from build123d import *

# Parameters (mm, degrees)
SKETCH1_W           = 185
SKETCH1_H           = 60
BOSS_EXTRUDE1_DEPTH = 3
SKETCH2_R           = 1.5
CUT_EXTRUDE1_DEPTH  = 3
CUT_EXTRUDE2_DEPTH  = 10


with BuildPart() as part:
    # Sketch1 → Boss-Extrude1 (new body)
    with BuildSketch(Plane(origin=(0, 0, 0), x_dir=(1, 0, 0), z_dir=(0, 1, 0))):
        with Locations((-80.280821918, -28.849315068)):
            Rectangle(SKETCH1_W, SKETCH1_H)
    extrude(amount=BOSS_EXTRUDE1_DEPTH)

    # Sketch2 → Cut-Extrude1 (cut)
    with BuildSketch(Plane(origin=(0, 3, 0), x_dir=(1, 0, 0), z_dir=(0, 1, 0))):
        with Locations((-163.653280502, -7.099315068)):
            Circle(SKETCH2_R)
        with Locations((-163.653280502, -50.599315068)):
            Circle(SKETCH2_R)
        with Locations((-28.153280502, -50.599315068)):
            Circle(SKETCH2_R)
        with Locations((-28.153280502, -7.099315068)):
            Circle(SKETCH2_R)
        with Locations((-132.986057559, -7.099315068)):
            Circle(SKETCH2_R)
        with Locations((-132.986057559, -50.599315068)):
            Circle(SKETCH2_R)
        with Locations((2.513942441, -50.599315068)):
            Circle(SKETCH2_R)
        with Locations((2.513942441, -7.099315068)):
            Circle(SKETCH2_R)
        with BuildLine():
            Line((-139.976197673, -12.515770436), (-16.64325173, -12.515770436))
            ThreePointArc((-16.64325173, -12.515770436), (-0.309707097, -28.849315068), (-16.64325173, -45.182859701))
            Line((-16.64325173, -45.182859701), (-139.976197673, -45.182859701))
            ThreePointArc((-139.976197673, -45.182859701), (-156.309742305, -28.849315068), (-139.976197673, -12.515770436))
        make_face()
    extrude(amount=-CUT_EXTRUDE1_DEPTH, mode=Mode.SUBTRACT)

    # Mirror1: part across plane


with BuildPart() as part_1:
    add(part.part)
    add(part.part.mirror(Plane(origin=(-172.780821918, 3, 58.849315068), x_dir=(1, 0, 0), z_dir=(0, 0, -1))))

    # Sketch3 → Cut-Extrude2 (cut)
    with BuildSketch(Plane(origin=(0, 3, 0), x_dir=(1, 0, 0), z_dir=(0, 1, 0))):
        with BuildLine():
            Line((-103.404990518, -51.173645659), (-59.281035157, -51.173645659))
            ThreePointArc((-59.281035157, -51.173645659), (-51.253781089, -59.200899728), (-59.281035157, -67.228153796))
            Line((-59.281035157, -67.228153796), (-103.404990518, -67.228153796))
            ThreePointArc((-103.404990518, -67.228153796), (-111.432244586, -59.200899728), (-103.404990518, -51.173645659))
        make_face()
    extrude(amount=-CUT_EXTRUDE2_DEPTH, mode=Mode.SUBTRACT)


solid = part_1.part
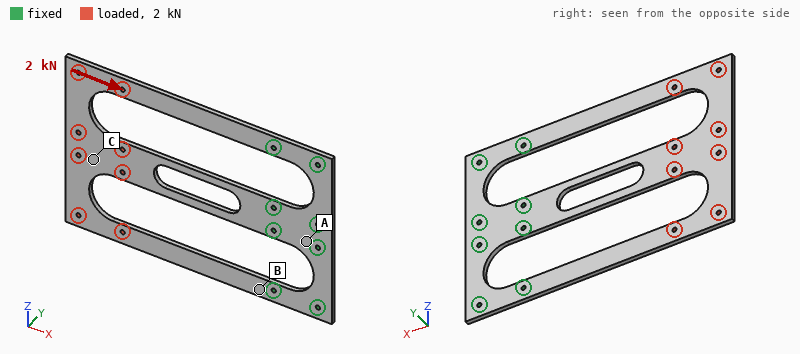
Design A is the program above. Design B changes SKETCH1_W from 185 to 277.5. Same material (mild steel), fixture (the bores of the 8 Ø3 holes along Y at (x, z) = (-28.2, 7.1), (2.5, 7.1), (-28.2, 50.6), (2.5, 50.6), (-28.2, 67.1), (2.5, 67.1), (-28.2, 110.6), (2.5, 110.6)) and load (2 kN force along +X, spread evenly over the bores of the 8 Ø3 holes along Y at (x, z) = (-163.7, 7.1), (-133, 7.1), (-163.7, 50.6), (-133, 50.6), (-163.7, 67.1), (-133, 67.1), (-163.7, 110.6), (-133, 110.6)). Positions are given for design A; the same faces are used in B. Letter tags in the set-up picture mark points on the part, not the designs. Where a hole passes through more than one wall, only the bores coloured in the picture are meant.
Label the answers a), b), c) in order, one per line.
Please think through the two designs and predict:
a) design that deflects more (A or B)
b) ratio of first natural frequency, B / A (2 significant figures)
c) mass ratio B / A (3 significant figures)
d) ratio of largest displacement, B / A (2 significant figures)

a) A
b) 0.50
c) 1.97
d) 0.83
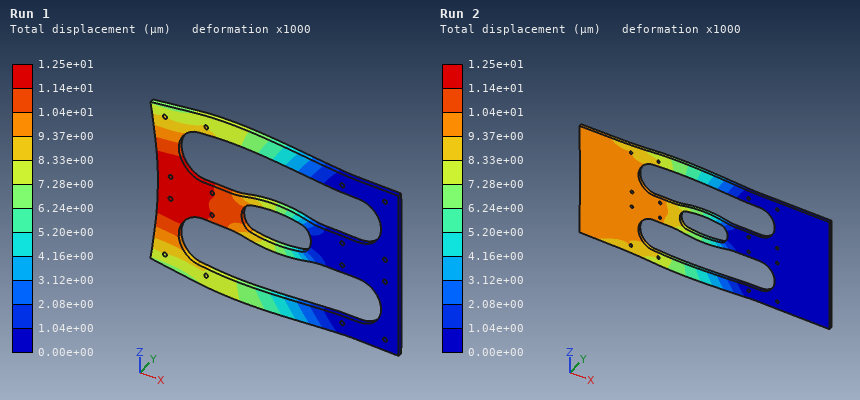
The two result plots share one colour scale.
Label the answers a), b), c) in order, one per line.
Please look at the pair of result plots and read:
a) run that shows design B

a) Run 2
